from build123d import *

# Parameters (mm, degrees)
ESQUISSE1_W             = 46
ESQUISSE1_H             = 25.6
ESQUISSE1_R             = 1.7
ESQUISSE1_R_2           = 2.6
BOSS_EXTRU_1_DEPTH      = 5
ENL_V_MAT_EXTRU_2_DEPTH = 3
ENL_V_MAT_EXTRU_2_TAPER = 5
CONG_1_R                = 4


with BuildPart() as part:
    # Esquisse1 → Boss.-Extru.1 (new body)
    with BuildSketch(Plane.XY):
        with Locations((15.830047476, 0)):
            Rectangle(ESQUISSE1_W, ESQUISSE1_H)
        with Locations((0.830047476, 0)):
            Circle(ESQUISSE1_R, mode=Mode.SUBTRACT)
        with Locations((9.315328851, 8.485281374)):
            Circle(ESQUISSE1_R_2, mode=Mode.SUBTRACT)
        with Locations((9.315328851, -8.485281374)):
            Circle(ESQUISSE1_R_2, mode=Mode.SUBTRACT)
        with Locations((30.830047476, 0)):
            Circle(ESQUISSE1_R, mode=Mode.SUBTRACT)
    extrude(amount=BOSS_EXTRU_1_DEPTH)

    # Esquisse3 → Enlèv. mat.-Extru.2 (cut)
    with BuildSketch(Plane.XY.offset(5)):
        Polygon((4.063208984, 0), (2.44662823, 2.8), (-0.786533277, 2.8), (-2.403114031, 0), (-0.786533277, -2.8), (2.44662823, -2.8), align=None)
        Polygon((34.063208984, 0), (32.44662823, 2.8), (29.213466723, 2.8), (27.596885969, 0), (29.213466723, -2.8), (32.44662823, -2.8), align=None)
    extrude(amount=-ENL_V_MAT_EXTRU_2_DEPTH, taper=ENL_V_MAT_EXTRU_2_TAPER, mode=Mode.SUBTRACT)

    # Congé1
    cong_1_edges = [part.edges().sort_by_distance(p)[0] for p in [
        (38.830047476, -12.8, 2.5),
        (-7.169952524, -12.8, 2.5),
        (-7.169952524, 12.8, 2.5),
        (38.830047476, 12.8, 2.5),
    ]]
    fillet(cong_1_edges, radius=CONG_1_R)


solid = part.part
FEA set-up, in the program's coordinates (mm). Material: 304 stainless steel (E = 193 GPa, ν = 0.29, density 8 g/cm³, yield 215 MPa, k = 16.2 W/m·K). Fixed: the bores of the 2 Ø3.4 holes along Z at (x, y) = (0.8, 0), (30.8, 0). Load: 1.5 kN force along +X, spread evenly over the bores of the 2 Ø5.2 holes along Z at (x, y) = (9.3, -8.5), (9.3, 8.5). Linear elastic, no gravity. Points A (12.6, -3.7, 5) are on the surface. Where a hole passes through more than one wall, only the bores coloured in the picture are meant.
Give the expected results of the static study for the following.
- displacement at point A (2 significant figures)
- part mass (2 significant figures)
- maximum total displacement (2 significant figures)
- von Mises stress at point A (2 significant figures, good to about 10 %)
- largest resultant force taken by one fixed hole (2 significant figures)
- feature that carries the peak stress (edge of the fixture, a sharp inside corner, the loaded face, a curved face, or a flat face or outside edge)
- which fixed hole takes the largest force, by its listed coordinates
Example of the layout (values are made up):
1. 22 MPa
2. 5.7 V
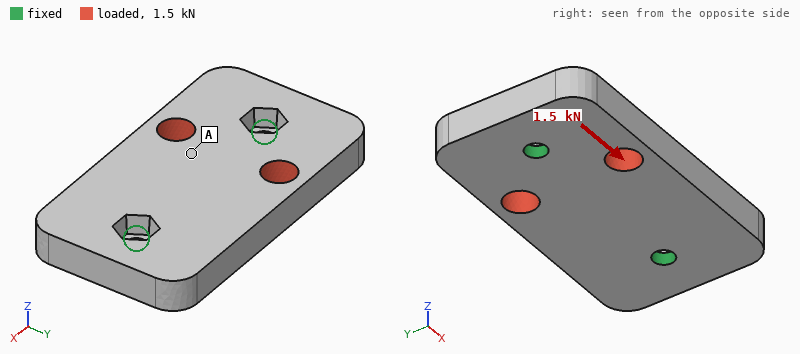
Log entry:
1. 0.95 µm
2. 43 g
3. 1.8 µm
4. 6.8 MPa
5. 840 N
6. edge of the fixture
7. (0.8, 0)
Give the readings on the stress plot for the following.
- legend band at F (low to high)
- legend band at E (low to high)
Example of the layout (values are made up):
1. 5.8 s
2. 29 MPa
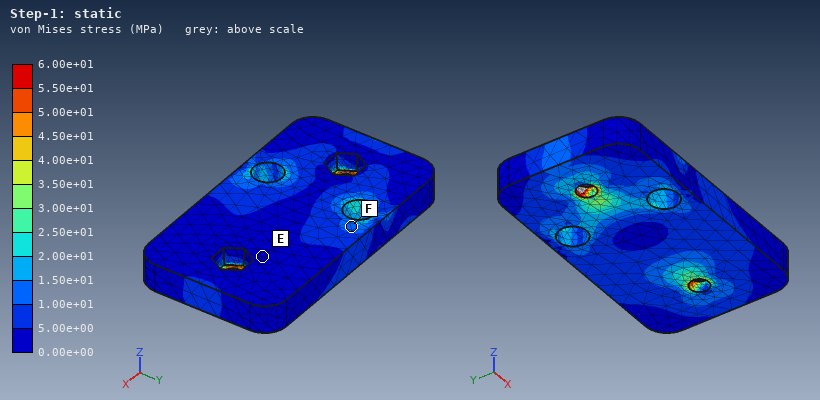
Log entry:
1. 1.00e+01 to 1.50e+01 MPa
2. 0.00e+00 to 5.00e+00 MPa
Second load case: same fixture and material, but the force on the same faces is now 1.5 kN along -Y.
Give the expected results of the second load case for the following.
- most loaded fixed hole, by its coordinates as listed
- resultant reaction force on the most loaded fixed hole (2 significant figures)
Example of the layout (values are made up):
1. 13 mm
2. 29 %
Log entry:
1. (0.8, 0)
2. 1.1 kN
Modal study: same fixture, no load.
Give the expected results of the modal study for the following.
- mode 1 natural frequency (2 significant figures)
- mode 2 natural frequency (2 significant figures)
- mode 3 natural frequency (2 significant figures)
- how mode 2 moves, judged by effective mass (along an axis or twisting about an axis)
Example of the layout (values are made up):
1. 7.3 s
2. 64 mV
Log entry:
1. 7200 Hz
2. 14 kHz
3. 14 kHz
4. along Z
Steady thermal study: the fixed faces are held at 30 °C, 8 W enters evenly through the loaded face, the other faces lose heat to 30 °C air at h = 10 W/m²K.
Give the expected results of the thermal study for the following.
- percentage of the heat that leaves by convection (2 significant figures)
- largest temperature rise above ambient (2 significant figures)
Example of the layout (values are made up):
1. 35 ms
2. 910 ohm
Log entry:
1. 8.4 %
2. 47 K
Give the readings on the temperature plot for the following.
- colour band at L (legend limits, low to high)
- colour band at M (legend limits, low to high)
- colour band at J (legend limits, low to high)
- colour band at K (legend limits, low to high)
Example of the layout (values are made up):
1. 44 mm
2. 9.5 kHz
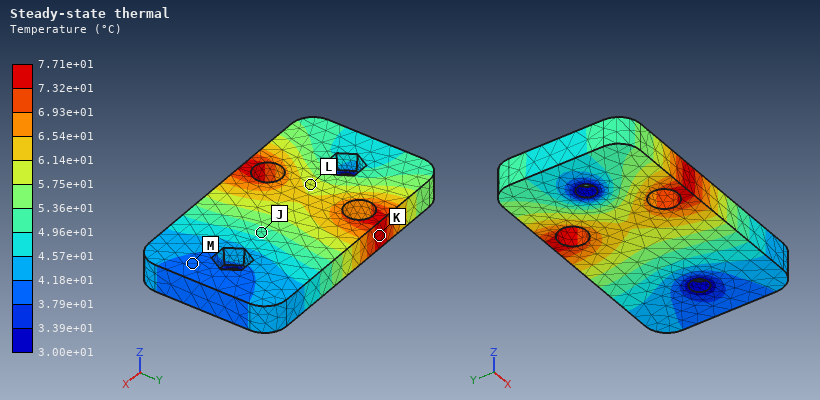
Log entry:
1. 5.75e+01 to 6.14e+01 °C
2. 3.79e+01 to 4.18e+01 °C
3. 4.96e+01 to 5.36e+01 °C
4. 7.32e+01 to 7.71e+01 °C
